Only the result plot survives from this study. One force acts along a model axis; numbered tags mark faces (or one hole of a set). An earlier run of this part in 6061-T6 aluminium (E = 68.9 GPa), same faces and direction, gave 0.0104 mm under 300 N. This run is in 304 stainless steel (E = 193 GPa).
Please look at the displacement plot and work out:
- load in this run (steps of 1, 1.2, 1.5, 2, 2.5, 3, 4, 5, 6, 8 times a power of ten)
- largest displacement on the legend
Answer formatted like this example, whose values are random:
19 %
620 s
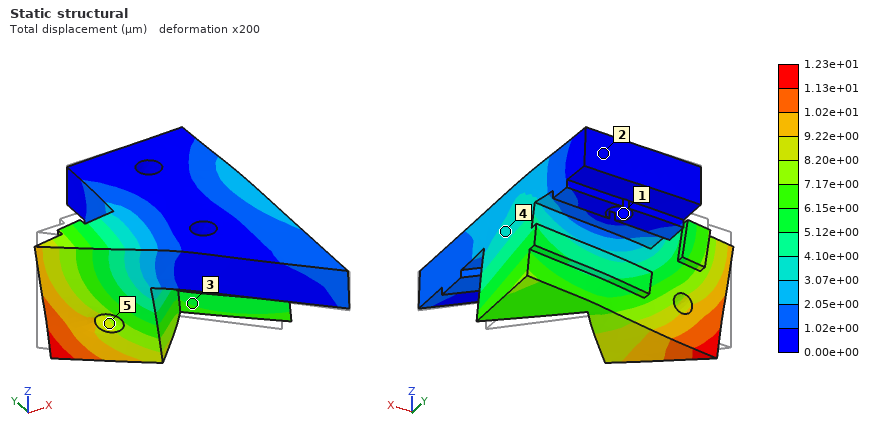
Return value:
1 kN
1.23e+01 µm
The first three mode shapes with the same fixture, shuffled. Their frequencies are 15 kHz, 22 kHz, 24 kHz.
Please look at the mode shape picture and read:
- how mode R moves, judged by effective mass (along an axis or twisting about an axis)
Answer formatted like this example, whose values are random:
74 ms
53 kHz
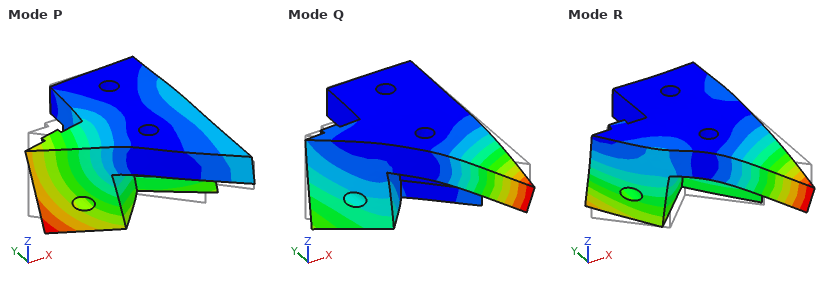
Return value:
along Y
